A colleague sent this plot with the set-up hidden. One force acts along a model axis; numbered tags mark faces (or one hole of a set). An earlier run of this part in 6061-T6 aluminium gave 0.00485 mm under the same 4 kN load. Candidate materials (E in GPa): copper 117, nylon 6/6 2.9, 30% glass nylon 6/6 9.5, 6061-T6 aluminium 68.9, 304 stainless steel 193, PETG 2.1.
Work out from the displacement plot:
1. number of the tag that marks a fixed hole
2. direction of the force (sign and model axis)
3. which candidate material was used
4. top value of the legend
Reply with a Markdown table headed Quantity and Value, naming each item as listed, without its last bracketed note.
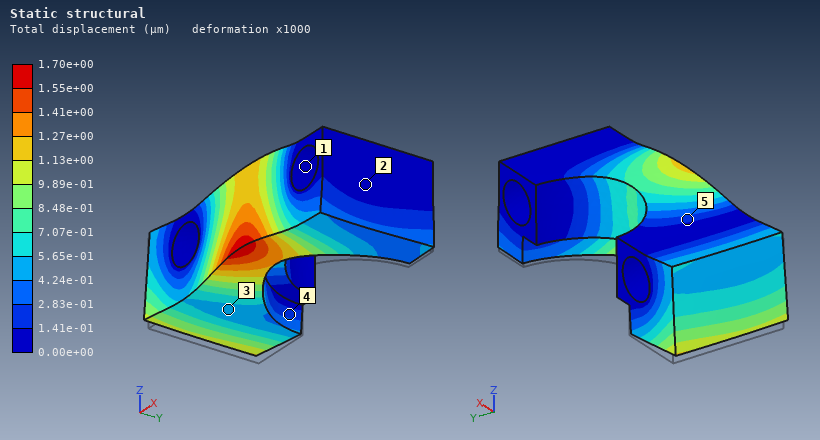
| Quantity | Value |
|---|---|
| number of the tag that marks a fixed hole | 1 |
| direction of the force | +Z |
| which candidate material was used | 304 stainless steel |
| top value of the legend | 1.70e+00 µm |
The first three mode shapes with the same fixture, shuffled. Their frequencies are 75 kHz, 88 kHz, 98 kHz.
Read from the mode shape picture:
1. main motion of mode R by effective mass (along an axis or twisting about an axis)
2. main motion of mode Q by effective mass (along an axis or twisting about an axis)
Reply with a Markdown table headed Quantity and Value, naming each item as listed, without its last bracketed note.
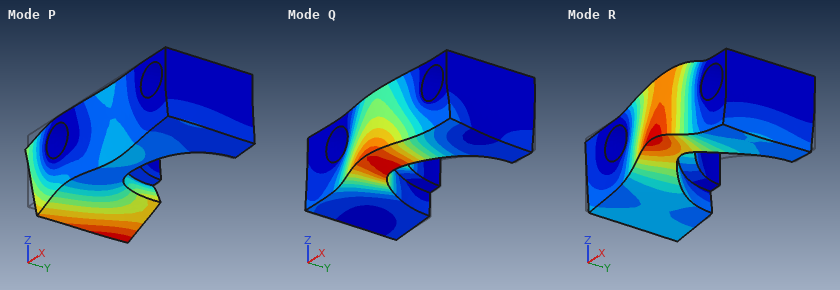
| Quantity | Value |
|---|---|
| main motion of mode R by effective mass | along Z |
| main motion of mode Q by effective mass | along Y |
